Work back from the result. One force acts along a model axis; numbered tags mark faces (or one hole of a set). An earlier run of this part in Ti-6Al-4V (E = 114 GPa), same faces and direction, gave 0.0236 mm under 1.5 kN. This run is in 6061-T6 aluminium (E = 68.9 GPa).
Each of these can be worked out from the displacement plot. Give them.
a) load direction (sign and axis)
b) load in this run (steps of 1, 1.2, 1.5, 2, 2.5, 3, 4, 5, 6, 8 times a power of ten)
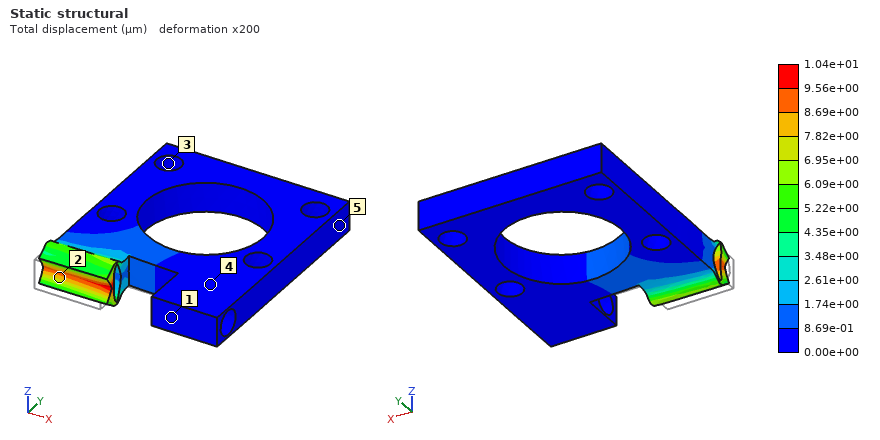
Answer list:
+Y
400 N
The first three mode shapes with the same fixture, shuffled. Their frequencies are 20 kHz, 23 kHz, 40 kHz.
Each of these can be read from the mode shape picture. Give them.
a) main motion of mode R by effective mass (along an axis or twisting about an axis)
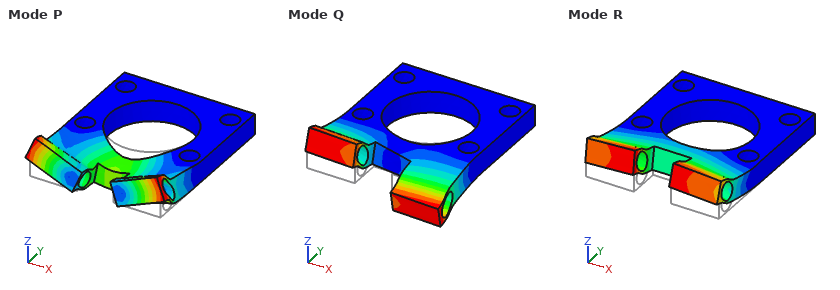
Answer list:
along Z
